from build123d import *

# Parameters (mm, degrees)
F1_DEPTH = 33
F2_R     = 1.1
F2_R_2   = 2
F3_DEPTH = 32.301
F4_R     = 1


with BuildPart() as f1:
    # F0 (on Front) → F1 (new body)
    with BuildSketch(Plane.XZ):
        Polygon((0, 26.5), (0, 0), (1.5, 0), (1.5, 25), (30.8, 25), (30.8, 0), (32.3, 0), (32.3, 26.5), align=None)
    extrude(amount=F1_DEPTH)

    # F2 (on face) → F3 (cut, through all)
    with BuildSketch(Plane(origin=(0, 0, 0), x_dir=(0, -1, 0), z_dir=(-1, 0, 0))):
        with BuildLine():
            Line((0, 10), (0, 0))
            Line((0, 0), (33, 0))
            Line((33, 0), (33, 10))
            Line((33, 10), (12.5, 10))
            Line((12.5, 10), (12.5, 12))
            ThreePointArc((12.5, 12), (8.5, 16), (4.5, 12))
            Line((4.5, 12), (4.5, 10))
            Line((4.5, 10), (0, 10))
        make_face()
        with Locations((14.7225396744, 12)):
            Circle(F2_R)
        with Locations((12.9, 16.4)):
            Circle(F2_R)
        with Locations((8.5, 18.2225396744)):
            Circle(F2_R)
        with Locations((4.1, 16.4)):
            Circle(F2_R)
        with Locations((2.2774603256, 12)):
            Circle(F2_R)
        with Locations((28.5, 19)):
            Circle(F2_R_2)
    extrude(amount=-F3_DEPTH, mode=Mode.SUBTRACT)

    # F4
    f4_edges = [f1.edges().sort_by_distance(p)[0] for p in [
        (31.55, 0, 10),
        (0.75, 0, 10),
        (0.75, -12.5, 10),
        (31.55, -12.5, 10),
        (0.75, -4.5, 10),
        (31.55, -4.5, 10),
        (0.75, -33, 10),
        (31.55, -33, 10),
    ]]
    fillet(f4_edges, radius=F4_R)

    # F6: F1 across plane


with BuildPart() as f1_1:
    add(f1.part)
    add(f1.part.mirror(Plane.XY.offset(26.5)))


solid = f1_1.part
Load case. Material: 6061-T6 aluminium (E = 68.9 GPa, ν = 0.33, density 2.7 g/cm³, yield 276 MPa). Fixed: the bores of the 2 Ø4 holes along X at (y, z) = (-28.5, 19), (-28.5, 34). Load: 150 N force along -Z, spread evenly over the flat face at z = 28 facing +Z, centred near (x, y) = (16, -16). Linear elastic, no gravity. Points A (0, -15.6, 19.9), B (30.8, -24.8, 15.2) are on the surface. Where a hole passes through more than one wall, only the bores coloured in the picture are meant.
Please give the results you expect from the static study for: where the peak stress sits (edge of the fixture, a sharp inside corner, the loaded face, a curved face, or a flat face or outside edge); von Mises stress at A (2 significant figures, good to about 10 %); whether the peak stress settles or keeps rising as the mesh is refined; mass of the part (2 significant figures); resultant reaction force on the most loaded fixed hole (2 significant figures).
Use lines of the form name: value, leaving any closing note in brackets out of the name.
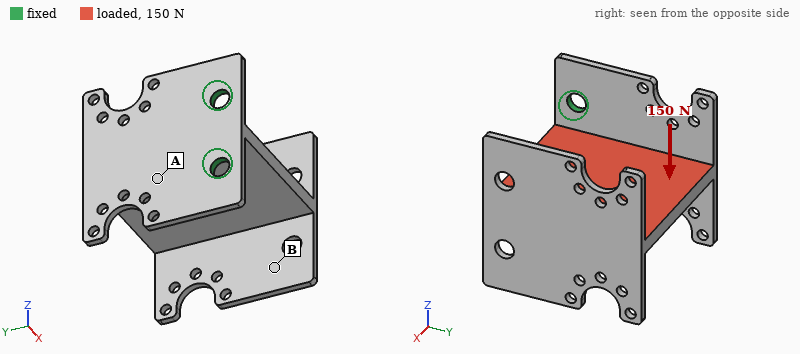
where the peak stress sits: edge of the fixture
von Mises stress at A: 38 MPa
whether the peak stress settles or keeps rising as the mesh is refined: keeps rising
mass of the part: 15 g
resultant reaction force on the most loaded fixed hole: 250 N
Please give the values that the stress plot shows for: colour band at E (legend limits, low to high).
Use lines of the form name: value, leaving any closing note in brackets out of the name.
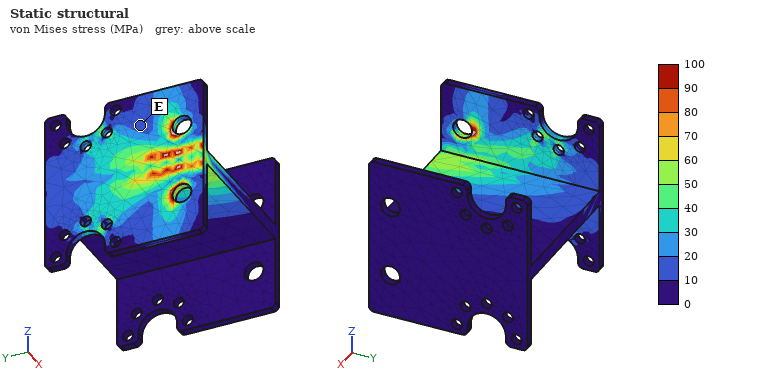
colour band at E: 10 to 20 MPa
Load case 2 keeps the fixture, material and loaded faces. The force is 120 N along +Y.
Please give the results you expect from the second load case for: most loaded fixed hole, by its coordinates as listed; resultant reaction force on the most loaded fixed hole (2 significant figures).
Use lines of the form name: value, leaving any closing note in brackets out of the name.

most loaded fixed hole, by its coordinates as listed: (-28.5, 34)
resultant reaction force on the most loaded fixed hole: 73 N
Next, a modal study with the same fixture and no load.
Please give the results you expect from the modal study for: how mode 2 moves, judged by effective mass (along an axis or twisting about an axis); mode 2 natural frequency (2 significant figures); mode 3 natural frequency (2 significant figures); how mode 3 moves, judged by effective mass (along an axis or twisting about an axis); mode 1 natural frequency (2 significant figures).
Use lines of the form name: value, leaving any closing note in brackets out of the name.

how mode 2 moves, judged by effective mass: along Z
mode 2 natural frequency: 940 Hz
mode 3 natural frequency: 2800 Hz
how mode 3 moves, judged by effective mass: twisting about X
mode 1 natural frequency: 910 Hz
